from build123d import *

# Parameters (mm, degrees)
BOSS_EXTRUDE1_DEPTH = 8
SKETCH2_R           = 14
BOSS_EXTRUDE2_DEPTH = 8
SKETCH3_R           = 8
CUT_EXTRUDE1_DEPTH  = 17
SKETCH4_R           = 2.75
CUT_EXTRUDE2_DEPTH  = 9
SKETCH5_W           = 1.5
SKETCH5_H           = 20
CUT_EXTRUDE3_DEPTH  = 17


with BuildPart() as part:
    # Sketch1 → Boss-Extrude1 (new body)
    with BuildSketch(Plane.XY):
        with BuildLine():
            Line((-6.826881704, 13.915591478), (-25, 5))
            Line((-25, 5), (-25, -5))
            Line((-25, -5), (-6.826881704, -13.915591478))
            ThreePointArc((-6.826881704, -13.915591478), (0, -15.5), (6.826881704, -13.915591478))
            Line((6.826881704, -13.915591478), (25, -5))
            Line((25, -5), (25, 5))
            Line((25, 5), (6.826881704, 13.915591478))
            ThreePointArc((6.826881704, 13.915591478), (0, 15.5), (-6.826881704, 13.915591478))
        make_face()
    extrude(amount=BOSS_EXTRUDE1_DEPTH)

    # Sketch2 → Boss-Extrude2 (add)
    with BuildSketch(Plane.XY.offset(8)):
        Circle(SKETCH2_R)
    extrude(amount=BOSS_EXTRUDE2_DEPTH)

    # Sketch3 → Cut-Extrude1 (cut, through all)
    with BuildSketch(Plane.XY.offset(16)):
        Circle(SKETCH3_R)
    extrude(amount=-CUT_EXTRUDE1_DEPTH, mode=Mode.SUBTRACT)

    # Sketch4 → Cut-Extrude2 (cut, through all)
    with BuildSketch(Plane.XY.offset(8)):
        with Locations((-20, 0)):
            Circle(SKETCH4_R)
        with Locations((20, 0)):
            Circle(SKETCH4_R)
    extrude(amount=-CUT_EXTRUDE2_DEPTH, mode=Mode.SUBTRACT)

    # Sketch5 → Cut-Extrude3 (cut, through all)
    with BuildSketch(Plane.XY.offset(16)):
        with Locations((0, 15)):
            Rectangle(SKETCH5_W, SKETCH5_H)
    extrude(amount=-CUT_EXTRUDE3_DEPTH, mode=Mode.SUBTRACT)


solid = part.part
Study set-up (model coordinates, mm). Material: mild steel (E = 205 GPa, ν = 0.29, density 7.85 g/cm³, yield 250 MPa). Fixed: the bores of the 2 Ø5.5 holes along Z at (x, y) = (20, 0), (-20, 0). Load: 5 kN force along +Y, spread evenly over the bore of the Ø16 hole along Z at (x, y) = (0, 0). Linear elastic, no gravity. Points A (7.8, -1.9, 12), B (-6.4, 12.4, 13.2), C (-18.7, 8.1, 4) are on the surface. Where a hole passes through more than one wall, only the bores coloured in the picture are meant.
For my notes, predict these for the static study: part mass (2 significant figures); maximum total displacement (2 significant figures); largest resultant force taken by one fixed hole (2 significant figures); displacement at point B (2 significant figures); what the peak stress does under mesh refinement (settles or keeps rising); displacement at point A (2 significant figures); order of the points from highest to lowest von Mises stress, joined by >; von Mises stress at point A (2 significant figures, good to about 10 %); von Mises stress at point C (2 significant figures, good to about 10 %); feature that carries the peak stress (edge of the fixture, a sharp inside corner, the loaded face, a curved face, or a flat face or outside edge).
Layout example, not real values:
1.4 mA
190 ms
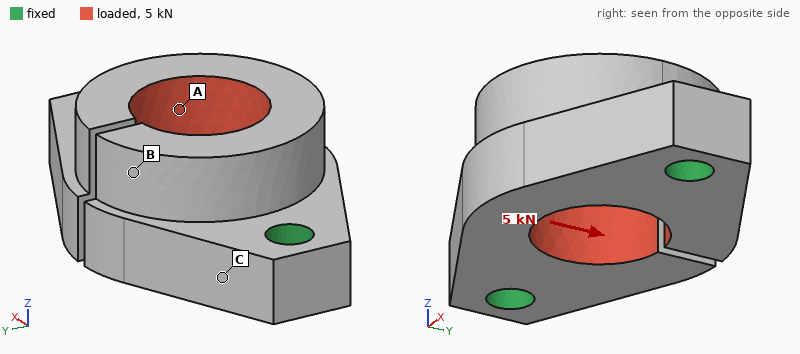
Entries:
78 g
19 µm
3.1 kN
14 µm
keeps rising
8.4 µm
C > A > B
25 MPa
53 MPa
edge of the fixture
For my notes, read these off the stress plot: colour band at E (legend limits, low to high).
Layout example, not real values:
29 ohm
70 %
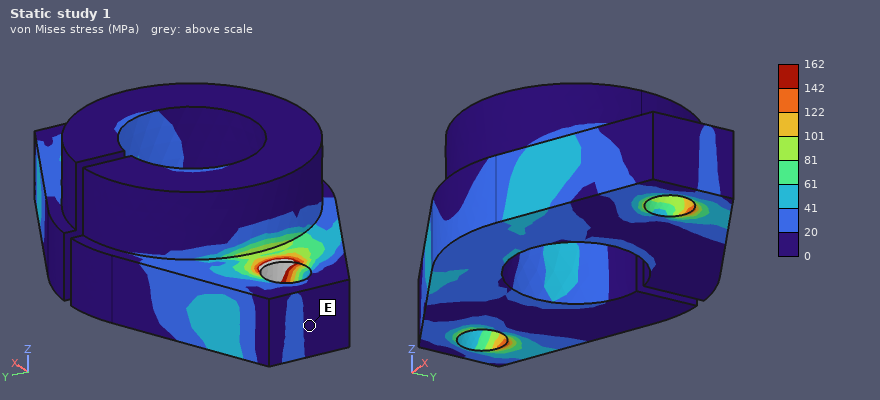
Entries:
0 to 20 MPa
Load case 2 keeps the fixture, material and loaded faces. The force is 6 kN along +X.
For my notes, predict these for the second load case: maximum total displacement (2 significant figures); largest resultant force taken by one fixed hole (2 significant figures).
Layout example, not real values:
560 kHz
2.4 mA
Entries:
10 µm
3.0 kN
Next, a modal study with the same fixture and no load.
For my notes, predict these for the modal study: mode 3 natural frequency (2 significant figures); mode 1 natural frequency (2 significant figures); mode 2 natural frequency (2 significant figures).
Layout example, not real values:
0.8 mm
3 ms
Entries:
14 kHz
13 kHz
13 kHz
